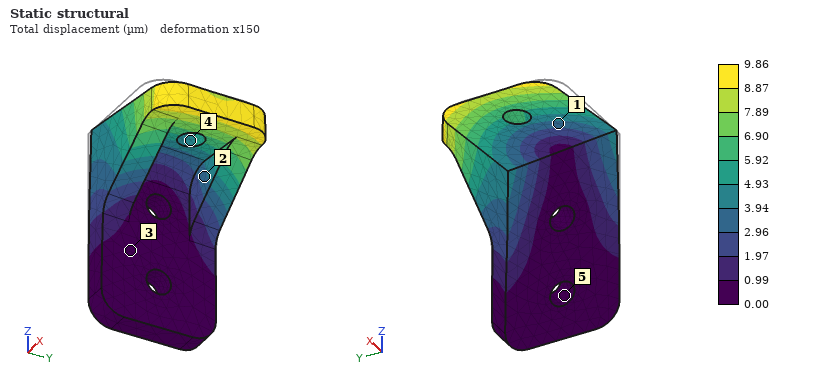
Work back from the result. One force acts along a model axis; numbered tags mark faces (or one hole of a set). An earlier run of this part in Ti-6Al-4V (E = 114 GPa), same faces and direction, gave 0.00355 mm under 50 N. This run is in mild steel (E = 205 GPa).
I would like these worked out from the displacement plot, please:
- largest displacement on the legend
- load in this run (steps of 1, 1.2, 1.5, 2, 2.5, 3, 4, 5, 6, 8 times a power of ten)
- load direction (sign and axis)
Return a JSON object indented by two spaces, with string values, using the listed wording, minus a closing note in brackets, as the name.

{
  "largest displacement on the legend": "9.86 µm",
  "load in this run": "250 N",
  "load direction": "+Y"
}
